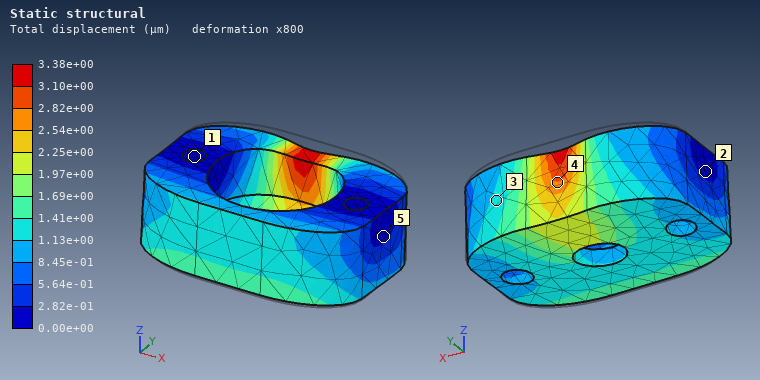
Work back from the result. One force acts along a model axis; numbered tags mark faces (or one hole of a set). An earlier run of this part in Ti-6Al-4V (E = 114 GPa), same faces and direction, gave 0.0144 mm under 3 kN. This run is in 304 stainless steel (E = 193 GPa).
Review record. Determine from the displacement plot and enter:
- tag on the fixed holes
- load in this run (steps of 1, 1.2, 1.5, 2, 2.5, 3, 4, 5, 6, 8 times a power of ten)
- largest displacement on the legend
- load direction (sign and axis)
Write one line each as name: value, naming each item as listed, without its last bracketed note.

tag on the fixed holes: 1
load in this run: 1.2 kN
largest displacement on the legend: 3.38e+00 µm
load direction: -Y
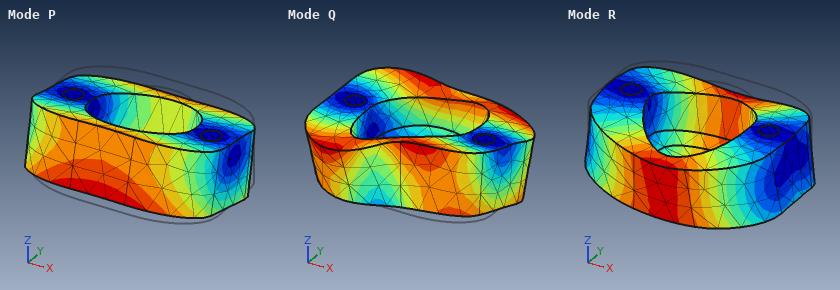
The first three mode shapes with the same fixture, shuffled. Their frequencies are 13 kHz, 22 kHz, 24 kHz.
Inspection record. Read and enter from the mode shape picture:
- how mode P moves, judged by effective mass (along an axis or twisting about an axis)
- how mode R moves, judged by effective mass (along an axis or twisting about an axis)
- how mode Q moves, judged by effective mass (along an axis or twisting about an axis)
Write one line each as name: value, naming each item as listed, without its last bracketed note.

how mode P moves, judged by effective mass: along Y
how mode R moves, judged by effective mass: along Z
how mode Q moves, judged by effective mass: twisting about Z
